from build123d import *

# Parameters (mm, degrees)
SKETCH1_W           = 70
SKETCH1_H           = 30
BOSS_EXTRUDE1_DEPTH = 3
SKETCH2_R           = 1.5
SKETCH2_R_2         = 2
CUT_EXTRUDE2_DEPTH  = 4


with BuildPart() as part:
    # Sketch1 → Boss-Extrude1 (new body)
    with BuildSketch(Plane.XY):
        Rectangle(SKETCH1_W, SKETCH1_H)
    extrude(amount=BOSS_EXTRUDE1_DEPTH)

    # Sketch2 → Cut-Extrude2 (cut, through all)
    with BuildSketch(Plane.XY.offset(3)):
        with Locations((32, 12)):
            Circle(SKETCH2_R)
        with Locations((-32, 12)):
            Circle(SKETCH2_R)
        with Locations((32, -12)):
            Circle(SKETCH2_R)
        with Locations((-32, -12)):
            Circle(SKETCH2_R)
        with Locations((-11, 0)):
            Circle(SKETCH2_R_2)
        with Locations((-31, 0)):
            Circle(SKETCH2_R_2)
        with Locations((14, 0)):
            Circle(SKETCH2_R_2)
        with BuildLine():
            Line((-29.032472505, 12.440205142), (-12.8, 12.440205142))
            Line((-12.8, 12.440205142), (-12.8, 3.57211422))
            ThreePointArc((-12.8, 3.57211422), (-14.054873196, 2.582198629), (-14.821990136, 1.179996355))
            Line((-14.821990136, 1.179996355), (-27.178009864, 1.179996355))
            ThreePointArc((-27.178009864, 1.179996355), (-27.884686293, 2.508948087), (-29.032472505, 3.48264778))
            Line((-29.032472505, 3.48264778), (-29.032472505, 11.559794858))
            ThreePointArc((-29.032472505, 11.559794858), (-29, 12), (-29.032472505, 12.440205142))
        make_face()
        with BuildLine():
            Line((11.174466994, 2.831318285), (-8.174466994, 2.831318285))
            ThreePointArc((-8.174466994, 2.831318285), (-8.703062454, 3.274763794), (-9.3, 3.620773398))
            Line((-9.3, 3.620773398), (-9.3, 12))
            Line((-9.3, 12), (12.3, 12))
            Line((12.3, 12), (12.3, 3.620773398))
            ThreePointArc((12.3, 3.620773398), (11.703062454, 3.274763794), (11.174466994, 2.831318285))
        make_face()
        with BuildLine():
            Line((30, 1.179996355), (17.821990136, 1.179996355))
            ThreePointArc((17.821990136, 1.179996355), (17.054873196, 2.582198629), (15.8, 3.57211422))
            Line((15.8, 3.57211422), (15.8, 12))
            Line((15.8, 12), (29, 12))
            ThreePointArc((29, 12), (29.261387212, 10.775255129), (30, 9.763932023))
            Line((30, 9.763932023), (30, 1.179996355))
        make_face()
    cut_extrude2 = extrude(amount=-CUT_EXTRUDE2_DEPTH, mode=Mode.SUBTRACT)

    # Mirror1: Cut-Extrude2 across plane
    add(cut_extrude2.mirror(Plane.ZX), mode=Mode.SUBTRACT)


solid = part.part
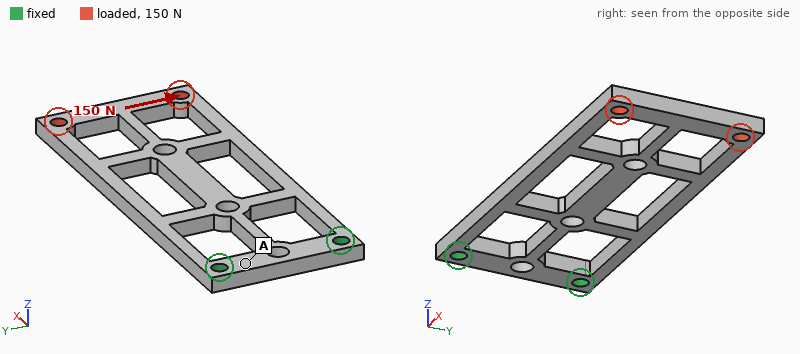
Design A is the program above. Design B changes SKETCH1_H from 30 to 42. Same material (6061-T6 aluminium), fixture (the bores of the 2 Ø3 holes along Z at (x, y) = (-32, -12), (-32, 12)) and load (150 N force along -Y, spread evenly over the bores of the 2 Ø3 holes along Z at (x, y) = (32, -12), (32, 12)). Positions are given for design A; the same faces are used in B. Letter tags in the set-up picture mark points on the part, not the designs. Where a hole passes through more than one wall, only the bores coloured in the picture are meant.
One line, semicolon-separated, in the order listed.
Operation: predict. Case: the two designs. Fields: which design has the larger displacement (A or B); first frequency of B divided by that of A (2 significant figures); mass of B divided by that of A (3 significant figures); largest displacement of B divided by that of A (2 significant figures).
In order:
A; 1.1; 1.85; 0.45
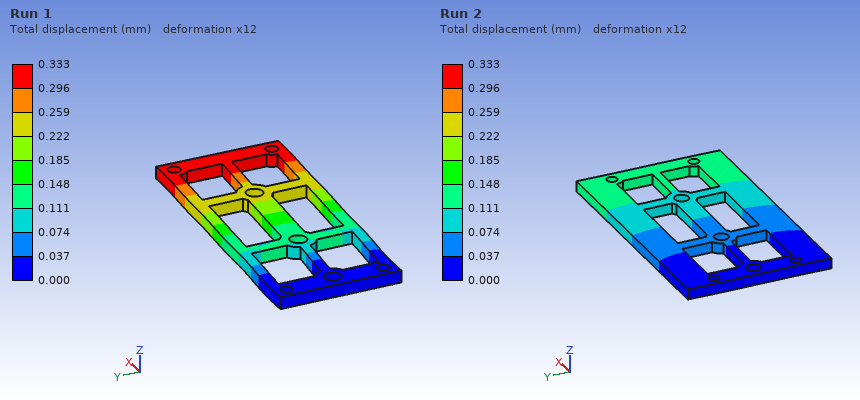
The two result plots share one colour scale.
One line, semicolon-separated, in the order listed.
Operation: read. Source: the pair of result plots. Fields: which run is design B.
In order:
Run 2
